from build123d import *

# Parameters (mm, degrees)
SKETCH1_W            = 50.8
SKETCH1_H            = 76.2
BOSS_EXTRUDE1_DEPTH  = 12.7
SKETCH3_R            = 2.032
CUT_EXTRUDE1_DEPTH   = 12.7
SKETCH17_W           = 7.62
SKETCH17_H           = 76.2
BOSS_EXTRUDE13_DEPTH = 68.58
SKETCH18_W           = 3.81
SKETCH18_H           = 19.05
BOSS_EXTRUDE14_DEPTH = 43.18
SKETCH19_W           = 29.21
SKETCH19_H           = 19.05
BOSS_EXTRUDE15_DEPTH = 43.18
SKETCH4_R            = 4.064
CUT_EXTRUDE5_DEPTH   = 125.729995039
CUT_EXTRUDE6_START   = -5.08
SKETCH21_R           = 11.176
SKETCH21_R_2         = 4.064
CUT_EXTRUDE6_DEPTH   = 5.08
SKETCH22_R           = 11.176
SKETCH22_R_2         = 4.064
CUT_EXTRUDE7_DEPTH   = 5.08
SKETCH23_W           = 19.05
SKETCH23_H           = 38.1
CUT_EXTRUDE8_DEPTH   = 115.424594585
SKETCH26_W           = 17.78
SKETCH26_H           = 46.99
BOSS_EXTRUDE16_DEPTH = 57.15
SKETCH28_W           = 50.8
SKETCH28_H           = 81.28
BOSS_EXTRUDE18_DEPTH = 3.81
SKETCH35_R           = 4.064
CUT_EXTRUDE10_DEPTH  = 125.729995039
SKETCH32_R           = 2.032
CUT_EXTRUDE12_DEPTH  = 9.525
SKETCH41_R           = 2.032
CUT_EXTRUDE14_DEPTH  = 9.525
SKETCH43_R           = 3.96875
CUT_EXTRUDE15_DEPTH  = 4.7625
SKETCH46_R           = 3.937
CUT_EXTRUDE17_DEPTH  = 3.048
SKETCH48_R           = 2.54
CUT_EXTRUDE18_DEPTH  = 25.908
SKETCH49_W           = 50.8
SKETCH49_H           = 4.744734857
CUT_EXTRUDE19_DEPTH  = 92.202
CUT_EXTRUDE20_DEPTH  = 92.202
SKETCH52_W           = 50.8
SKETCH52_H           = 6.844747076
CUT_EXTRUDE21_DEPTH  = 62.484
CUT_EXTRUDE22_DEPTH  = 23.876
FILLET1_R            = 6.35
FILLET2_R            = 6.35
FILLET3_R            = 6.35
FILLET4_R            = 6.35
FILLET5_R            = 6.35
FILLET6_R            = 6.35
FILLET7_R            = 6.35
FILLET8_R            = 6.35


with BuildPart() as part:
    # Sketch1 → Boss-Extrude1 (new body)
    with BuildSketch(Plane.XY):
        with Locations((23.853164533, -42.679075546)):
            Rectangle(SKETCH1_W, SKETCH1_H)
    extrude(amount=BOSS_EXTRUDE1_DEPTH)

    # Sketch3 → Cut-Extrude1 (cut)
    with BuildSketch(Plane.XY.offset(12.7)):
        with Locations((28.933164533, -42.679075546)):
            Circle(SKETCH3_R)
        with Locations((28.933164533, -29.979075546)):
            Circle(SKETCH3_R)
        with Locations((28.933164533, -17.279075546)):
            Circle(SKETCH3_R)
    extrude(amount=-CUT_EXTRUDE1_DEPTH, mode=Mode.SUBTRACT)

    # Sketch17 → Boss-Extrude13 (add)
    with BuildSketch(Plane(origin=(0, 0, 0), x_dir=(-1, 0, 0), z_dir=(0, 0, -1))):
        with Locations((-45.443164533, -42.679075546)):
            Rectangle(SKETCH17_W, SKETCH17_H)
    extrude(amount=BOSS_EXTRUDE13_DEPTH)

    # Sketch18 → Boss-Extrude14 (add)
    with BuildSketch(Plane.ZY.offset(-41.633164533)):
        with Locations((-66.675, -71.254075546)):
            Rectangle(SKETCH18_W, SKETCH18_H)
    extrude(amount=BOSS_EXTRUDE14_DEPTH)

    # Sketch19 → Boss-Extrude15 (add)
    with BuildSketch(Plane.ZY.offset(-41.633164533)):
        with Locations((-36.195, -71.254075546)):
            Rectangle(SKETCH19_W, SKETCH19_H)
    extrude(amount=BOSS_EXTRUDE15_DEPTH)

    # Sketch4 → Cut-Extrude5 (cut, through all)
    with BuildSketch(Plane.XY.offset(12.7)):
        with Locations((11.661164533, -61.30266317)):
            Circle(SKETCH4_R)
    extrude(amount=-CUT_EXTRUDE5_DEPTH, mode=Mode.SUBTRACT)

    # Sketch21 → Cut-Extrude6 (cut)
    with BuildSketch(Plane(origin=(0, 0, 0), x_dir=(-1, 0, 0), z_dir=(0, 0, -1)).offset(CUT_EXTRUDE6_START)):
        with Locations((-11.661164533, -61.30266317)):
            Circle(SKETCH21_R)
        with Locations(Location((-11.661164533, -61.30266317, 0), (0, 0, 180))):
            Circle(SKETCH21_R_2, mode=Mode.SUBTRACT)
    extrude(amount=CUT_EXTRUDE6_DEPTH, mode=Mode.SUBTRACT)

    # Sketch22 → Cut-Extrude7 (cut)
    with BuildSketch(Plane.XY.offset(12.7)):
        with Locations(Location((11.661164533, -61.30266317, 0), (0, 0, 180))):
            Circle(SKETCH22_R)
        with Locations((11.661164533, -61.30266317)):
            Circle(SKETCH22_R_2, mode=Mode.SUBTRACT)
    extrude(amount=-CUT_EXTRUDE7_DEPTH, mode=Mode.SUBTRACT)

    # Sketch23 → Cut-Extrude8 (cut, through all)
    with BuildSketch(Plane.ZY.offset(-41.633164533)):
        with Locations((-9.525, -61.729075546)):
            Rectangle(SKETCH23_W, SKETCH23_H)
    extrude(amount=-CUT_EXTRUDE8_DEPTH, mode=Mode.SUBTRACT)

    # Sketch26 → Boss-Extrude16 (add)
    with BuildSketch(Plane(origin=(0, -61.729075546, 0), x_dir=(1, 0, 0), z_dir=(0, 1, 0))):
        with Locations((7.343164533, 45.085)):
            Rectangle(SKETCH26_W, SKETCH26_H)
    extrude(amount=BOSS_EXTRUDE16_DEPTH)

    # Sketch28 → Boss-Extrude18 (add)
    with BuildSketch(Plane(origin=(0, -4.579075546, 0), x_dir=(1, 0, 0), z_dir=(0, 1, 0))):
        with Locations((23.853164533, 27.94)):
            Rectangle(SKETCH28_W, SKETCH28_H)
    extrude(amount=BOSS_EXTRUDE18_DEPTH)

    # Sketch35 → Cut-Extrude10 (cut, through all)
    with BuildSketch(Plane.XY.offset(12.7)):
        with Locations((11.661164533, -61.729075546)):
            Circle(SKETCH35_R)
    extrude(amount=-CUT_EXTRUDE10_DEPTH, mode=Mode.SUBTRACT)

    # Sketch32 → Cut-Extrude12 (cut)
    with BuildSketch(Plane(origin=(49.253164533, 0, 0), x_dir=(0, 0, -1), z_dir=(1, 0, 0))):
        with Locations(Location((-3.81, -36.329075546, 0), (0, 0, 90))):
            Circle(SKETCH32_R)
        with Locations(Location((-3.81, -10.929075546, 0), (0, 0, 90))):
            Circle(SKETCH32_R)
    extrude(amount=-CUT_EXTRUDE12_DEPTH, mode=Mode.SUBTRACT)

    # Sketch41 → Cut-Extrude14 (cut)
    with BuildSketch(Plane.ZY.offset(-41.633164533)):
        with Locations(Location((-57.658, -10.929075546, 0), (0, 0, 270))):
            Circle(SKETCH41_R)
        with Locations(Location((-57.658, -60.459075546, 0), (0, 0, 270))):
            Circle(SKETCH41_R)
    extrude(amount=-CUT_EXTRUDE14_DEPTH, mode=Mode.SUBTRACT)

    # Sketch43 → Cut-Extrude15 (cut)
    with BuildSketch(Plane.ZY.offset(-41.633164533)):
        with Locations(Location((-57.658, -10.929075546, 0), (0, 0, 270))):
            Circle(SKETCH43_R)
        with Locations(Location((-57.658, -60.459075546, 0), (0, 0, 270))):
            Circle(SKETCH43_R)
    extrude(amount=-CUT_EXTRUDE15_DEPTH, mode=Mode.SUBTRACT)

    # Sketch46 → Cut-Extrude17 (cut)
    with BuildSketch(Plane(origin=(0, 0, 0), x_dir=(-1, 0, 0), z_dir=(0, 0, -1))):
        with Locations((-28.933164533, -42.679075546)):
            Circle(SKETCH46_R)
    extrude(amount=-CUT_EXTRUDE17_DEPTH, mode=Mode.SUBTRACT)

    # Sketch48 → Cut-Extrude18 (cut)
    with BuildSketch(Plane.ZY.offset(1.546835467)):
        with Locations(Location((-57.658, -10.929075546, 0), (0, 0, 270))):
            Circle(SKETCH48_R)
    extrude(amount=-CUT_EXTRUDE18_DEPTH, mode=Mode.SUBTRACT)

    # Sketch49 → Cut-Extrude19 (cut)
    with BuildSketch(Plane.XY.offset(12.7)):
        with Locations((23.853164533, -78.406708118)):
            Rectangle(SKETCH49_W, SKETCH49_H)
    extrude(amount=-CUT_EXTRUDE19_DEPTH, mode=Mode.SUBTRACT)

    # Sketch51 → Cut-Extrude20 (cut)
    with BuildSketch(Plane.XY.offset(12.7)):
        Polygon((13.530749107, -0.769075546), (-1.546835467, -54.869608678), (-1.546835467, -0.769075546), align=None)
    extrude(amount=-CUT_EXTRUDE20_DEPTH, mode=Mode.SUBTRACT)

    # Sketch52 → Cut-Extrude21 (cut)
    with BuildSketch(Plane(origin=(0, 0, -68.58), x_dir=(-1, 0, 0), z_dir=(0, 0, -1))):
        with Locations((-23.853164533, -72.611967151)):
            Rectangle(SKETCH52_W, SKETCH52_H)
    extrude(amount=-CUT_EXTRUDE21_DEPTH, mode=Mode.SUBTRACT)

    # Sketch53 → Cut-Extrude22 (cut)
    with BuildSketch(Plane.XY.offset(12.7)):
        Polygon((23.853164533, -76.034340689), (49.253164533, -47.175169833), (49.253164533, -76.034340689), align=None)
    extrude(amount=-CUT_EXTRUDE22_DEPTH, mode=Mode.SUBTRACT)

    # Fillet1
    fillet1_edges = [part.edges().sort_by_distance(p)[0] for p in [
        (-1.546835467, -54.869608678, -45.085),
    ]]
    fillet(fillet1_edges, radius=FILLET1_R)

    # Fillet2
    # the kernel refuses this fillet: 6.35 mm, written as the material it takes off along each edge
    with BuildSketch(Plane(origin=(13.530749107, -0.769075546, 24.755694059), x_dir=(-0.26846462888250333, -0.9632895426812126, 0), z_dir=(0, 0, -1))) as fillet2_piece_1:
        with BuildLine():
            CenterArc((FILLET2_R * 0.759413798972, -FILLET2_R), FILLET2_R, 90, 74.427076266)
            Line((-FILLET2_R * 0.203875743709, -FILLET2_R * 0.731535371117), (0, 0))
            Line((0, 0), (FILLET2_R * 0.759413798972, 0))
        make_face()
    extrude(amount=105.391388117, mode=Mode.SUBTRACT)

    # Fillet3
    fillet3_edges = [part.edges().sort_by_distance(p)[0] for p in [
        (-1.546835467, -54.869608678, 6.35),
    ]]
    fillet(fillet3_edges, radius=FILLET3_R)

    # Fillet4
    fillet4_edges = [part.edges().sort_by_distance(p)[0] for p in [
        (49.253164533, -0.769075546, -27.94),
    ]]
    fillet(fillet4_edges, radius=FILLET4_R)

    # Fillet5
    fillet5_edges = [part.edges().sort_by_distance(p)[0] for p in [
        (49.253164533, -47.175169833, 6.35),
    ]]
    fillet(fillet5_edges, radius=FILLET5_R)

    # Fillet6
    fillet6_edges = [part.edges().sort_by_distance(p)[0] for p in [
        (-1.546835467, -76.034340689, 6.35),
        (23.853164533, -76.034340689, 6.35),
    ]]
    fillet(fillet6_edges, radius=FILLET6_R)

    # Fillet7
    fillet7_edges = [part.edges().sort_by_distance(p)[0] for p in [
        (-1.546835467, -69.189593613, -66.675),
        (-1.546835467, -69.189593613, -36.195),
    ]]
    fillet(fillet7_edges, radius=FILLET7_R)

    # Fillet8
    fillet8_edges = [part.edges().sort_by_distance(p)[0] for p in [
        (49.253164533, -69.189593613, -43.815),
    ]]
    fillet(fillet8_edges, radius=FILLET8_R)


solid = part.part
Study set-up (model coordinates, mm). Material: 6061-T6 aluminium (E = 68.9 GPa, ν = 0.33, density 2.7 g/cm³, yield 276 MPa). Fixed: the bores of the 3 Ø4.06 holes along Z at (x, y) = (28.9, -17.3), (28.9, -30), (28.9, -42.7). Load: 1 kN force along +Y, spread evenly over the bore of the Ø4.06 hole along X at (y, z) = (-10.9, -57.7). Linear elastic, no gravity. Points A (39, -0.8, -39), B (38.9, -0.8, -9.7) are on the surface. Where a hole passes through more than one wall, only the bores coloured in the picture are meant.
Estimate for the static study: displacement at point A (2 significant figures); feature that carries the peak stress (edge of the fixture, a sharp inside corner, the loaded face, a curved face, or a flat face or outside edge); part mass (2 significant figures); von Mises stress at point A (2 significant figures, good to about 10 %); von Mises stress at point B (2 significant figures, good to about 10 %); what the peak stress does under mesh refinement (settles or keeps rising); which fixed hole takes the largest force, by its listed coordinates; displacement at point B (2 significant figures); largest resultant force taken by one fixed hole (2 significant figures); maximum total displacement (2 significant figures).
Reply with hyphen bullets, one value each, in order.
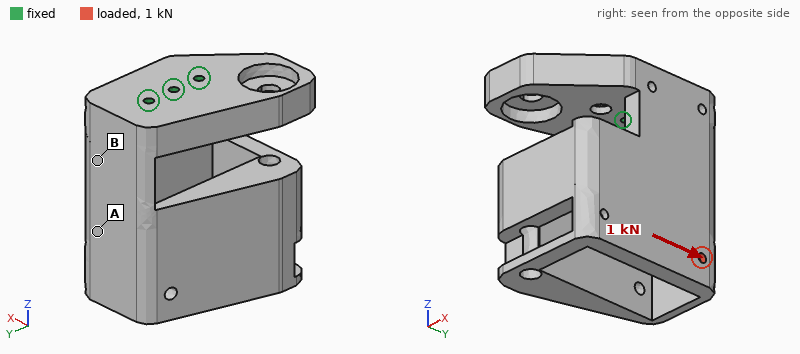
- 0.070 mm
- edge of the fixture
- 300 g
- 5.6 MPa
- 14 MPa
- keeps rising
- (28.9, -17.3)
- 0.028 mm
- 2.1 kN
- 0.16 mm
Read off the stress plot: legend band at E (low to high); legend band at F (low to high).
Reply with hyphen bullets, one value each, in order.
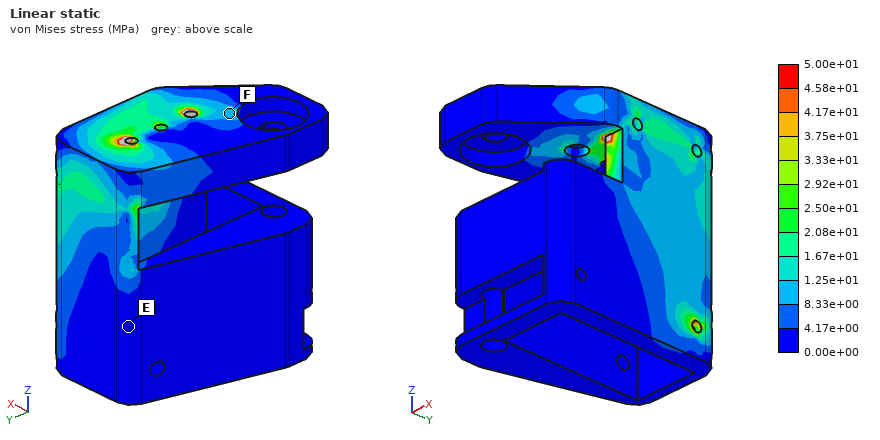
- 0.00e+00 to 4.17e+00 MPa
- 8.33e+00 to 1.25e+01 MPa
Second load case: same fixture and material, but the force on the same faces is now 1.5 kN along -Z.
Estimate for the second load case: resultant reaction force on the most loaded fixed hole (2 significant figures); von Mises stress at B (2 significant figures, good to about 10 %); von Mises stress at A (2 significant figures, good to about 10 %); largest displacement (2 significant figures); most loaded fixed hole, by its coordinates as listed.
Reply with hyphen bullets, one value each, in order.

- 1.4 kN
- 9.7 MPa
- 6.0 MPa
- 98 µm
- (28.9, -17.3)
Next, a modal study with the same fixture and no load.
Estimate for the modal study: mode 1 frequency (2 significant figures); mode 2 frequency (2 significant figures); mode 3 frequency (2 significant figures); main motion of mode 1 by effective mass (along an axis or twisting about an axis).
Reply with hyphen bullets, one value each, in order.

- 730 Hz
- 890 Hz
- 2200 Hz
- along X
